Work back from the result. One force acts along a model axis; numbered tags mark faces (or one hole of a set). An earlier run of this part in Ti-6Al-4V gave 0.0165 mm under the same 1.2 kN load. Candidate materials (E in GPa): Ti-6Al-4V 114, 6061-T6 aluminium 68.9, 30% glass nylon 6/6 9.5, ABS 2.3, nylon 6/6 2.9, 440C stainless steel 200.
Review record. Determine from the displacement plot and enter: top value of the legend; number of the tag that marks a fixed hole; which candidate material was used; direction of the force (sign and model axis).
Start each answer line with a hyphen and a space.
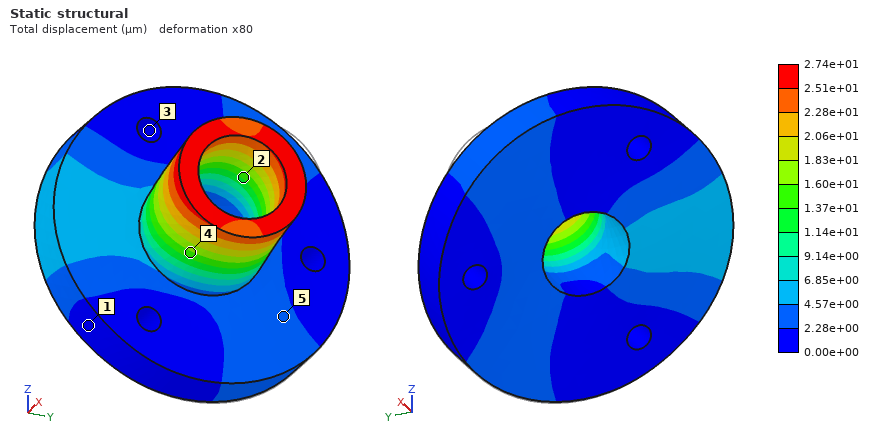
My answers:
- 2.74e+01 µm
- 3
- 6061-T6 aluminium
- -Y
